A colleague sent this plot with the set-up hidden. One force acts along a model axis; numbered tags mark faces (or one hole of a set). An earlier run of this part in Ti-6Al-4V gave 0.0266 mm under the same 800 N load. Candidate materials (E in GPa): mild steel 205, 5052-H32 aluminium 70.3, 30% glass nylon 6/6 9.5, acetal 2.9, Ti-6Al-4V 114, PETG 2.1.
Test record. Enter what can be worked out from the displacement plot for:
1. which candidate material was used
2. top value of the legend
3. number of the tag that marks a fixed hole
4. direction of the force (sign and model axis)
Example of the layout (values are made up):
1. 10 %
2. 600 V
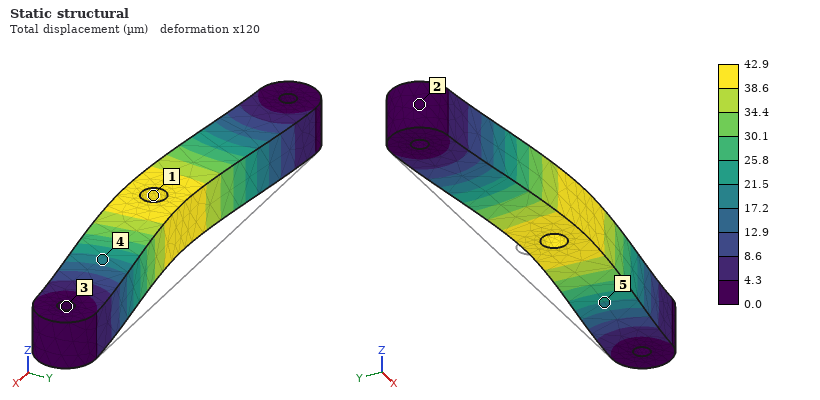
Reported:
1. 5052-H32 aluminium
2. 42.9 µm
3. 3
4. -Y
